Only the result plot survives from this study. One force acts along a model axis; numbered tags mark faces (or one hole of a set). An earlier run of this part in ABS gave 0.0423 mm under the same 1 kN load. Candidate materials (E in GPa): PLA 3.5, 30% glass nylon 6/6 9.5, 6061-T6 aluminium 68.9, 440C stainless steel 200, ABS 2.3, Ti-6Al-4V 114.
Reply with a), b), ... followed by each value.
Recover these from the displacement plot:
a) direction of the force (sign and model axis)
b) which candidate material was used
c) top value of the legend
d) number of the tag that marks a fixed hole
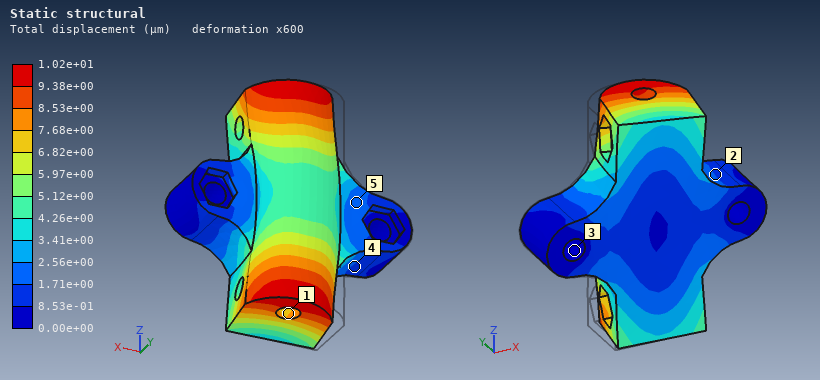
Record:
a) +X
b) 30% glass nylon 6/6
c) 1.02e+01 µm
d) 3
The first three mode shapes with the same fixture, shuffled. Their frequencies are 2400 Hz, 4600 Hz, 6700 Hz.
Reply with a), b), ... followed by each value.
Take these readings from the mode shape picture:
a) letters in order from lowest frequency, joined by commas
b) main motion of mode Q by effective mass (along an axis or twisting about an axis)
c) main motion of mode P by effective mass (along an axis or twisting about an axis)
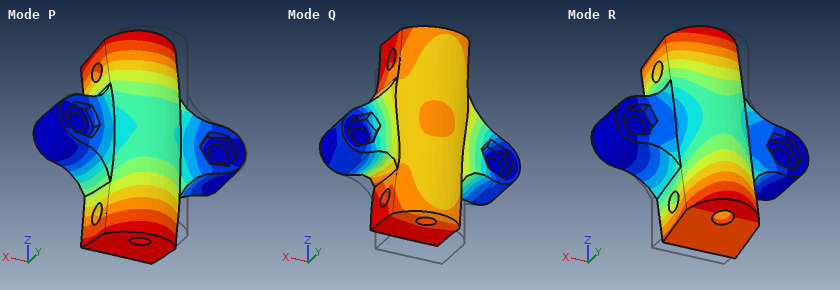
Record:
a) R, P, Q
b) along Z
c) along Y
